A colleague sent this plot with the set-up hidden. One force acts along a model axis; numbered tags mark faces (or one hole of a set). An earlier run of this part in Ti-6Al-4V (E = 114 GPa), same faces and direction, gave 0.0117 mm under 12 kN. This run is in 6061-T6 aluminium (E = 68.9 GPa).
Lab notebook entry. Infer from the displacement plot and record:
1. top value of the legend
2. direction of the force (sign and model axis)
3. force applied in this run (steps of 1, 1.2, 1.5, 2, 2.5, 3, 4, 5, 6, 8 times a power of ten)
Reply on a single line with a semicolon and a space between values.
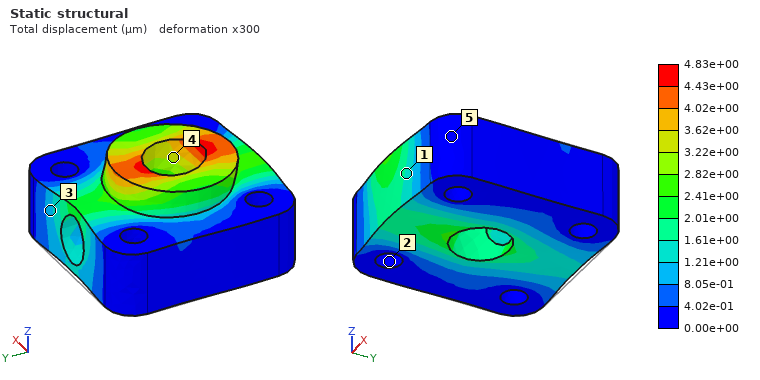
4.83e+00 µm; -Y; 3 kN
